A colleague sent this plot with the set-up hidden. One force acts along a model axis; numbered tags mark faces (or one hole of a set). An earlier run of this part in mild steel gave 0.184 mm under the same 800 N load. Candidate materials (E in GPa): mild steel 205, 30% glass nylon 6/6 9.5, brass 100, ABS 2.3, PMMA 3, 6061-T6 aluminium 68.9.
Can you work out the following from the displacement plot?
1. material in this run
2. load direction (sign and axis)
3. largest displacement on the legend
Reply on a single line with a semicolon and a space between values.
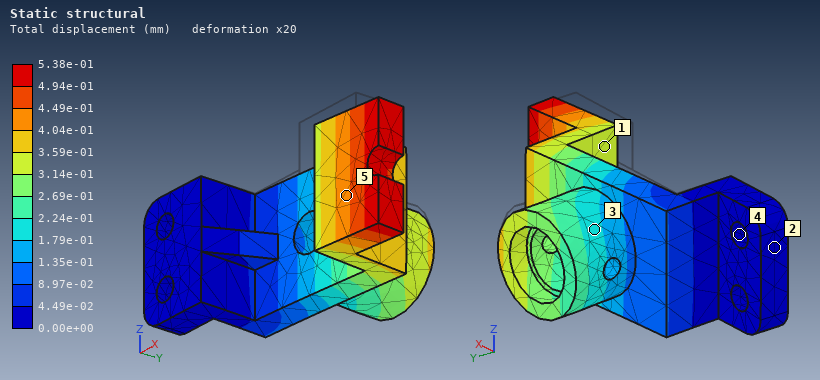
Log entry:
6061-T6 aluminium; +Y; 5.38e-01 mm
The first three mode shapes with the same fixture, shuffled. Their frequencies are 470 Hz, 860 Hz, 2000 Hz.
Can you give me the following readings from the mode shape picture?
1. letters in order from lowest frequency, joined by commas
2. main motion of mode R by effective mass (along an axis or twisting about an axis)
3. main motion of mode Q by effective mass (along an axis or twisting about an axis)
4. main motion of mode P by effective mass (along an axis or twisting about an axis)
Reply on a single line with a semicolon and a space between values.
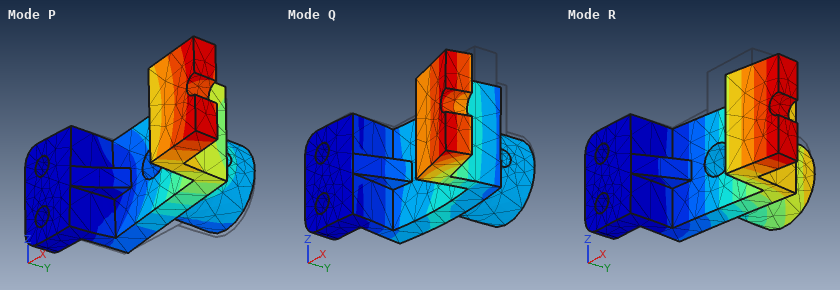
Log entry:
R, P, Q; along Y; along X; along Z
